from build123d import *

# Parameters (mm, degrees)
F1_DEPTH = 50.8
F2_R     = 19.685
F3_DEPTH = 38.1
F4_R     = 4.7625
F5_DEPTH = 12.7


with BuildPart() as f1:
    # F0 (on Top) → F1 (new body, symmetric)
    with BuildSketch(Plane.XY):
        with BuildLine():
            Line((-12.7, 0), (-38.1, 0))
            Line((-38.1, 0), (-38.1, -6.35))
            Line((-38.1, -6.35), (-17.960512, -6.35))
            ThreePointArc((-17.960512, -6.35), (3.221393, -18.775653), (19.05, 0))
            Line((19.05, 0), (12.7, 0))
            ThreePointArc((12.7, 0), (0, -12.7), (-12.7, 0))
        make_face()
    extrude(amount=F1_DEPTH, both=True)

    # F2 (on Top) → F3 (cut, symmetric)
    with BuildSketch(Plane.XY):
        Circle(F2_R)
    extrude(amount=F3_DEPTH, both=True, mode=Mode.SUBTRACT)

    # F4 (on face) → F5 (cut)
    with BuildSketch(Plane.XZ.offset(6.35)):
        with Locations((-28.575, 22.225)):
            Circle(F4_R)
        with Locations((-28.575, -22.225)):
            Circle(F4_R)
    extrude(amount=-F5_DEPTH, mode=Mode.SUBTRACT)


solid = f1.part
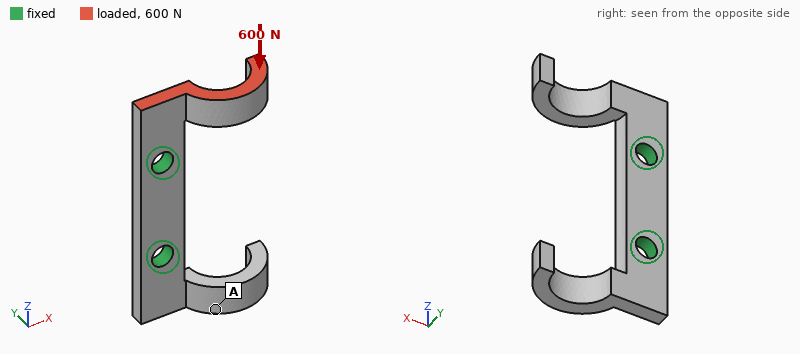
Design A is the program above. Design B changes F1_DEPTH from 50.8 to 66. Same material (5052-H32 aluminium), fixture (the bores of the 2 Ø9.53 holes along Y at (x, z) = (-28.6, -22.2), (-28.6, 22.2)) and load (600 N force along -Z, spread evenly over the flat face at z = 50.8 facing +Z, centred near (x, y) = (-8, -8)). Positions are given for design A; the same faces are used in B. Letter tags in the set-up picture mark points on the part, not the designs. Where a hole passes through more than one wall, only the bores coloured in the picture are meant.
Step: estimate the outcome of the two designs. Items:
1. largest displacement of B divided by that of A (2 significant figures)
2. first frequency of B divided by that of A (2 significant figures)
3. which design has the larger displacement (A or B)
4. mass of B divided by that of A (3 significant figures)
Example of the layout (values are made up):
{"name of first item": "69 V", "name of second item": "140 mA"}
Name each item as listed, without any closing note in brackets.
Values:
{"largest displacement of B divided by that of A": "0.61", "first frequency of B divided by that of A": "0.69", "which design has the larger displacement": "A", "mass of B divided by that of A": "1.69"}
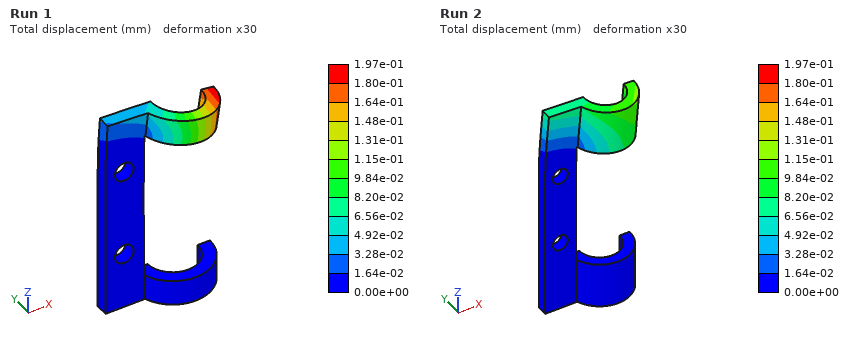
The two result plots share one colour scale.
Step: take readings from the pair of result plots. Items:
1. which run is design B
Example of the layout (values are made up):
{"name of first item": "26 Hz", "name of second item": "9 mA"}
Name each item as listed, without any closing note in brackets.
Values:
{"which run is design B": "Run 2"}
